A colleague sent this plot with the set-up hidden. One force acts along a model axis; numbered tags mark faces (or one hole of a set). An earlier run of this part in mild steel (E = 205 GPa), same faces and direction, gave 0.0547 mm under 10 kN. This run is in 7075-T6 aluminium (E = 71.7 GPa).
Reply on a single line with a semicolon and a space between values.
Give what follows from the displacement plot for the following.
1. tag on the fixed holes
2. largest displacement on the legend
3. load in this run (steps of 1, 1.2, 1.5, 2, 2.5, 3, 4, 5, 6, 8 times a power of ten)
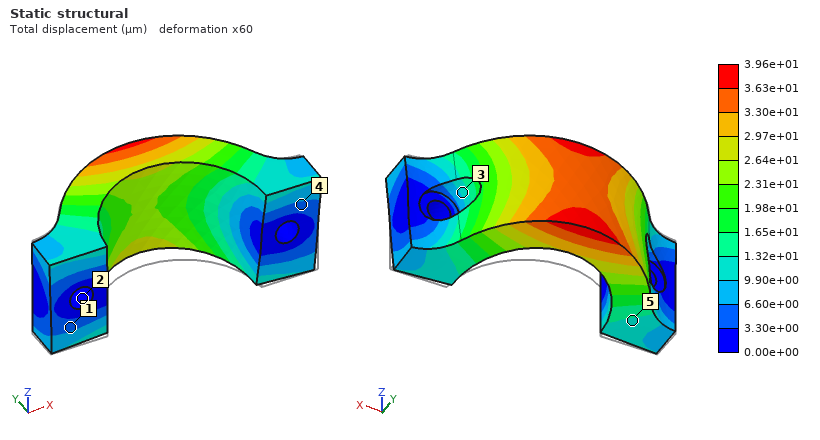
2; 3.96e+01 µm; 2.5 kN
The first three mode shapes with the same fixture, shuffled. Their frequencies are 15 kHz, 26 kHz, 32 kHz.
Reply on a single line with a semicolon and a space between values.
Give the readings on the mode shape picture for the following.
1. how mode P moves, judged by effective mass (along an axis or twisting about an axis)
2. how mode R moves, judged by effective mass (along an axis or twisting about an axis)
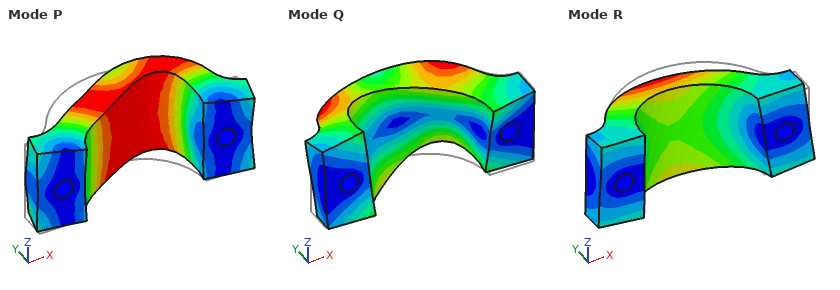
along X; along Z
